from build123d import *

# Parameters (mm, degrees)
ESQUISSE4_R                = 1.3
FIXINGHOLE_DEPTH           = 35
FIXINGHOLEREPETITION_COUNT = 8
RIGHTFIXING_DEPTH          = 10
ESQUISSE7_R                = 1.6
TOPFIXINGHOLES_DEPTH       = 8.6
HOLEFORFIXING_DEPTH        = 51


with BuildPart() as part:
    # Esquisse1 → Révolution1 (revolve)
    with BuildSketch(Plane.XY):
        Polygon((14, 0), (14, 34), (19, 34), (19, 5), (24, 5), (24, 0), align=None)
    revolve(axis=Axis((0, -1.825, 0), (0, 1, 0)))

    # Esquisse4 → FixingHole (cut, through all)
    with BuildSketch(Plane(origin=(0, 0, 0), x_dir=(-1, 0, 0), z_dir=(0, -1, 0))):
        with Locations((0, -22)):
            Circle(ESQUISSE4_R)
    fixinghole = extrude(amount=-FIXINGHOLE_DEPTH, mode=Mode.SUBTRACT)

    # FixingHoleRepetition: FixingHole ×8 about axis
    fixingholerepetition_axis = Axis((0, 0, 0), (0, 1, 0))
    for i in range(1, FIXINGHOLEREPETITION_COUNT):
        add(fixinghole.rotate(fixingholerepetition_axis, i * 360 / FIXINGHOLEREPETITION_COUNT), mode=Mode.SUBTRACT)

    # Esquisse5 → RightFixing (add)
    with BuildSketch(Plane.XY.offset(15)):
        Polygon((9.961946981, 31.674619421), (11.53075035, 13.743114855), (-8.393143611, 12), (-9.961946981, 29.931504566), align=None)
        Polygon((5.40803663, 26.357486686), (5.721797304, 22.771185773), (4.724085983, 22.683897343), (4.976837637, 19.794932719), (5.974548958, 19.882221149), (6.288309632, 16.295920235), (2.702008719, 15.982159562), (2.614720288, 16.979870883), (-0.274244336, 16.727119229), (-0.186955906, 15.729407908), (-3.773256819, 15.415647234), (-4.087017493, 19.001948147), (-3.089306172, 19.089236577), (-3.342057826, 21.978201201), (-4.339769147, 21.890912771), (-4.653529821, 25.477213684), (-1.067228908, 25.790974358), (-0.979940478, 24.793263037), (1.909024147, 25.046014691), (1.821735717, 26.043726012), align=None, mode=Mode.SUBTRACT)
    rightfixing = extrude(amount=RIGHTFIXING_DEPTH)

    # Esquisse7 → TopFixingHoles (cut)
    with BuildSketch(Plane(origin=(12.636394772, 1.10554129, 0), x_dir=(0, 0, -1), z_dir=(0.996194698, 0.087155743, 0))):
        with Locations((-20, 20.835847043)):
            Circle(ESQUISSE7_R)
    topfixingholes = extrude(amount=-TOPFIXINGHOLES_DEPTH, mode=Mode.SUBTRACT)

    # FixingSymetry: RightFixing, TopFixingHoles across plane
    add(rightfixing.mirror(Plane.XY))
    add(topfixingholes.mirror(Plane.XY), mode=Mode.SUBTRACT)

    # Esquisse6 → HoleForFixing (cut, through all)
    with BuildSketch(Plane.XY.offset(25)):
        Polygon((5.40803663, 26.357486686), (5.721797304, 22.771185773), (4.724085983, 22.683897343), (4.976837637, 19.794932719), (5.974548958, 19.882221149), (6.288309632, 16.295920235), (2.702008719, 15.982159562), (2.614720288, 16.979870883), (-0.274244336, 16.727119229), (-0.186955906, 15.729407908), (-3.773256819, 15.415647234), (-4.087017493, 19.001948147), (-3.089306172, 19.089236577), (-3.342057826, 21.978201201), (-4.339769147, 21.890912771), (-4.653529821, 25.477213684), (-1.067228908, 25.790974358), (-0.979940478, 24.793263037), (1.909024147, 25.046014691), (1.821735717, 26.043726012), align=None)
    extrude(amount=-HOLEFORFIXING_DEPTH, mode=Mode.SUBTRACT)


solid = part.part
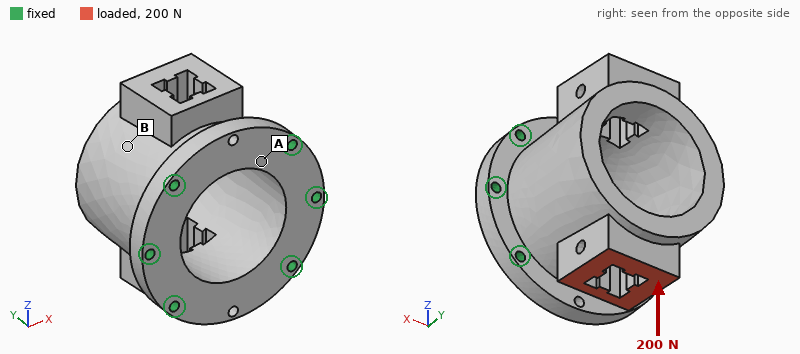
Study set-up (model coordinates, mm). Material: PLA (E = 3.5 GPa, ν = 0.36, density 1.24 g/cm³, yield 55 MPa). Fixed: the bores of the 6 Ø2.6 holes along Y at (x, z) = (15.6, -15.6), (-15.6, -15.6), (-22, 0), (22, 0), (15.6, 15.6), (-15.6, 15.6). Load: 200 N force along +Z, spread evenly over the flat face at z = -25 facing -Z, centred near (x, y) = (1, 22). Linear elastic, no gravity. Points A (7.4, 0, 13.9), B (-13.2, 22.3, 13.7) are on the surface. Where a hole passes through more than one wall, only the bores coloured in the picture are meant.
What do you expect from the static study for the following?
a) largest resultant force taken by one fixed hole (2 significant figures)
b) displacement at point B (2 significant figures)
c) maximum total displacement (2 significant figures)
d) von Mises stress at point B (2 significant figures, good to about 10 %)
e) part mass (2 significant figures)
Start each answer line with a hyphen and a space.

- 85 N
- 19 µm
- 59 µm
- 0.79 MPa
- 29 g
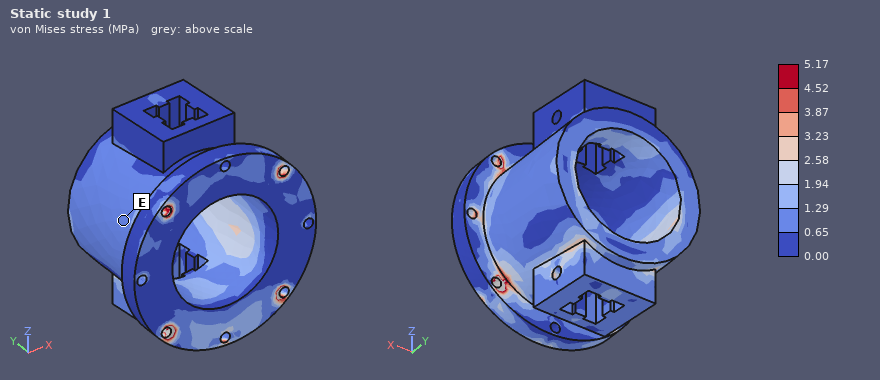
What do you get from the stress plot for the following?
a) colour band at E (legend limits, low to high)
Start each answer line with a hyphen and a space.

- 0.65 to 1.29 MPa
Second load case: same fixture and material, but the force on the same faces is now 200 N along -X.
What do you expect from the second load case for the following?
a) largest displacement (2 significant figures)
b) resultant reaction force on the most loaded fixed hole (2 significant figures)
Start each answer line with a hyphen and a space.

- 55 µm
- 74 N
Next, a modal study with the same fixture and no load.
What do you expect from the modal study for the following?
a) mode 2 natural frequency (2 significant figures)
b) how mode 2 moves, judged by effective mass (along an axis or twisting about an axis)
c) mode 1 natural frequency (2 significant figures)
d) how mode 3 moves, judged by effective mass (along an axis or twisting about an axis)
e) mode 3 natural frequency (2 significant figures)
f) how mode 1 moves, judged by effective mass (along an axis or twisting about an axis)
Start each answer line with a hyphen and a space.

- 3600 Hz
- along X
- 2900 Hz
- along Y
- 4300 Hz
- along Z
